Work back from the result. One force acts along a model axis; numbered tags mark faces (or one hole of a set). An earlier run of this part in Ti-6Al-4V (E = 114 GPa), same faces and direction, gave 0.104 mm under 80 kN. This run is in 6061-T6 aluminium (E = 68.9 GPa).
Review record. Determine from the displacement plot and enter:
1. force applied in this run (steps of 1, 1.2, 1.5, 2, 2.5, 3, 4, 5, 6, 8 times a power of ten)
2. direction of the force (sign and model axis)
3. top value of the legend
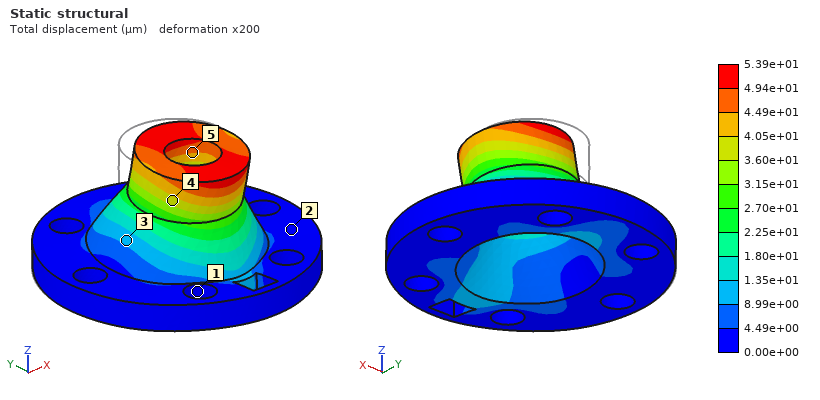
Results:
25 kN
-Y
5.39e+01 µm
